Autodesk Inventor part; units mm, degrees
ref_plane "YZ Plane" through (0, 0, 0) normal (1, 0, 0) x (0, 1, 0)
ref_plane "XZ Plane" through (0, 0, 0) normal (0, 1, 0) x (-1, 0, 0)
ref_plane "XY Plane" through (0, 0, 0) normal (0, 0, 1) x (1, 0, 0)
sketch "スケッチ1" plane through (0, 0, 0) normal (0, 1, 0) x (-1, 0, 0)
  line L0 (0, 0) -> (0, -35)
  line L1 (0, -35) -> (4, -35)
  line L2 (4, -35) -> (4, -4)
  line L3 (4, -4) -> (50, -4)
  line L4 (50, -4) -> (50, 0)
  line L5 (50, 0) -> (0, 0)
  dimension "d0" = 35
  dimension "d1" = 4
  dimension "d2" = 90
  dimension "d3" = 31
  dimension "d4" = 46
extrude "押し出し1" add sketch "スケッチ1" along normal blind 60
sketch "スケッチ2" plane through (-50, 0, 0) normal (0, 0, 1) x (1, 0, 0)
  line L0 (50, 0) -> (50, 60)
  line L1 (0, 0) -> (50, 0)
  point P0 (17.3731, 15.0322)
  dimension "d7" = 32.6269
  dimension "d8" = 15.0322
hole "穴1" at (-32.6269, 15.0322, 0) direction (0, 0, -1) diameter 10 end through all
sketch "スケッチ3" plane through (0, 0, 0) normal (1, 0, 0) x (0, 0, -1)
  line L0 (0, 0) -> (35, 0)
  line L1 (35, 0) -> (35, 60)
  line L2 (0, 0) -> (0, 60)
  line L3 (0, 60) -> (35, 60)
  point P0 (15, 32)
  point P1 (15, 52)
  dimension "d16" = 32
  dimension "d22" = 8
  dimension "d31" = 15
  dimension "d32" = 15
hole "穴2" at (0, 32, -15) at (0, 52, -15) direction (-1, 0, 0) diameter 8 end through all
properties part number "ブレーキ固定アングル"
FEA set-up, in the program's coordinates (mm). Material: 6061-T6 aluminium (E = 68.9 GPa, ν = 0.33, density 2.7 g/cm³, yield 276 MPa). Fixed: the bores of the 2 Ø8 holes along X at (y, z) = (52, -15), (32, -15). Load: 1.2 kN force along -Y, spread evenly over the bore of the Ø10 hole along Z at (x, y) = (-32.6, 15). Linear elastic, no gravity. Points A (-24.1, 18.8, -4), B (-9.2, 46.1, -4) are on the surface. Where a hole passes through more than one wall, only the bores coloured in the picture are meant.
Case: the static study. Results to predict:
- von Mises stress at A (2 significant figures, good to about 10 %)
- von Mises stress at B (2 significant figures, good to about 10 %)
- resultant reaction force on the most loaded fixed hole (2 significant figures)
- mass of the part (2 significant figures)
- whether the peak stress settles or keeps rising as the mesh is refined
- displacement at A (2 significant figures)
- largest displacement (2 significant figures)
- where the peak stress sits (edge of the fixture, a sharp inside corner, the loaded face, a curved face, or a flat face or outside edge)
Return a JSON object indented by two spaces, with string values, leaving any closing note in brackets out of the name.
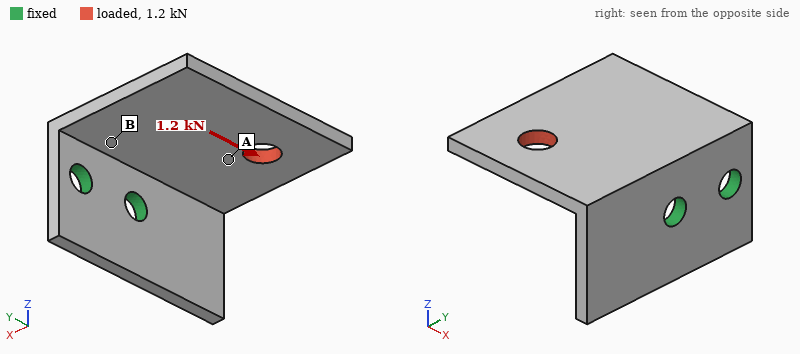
{
  "von Mises stress at A": "27 MPa",
  "von Mises stress at B": "59 MPa",
  "resultant reaction force on the most loaded fixed hole": "1.6 kN",
  "mass of the part": "51 g",
  "whether the peak stress settles or keeps rising as the mesh is refined": "keeps rising",
  "displacement at A": "0.14 mm",
  "largest displacement": "0.31 mm",
  "where the peak stress sits": "edge of the fixture"
}
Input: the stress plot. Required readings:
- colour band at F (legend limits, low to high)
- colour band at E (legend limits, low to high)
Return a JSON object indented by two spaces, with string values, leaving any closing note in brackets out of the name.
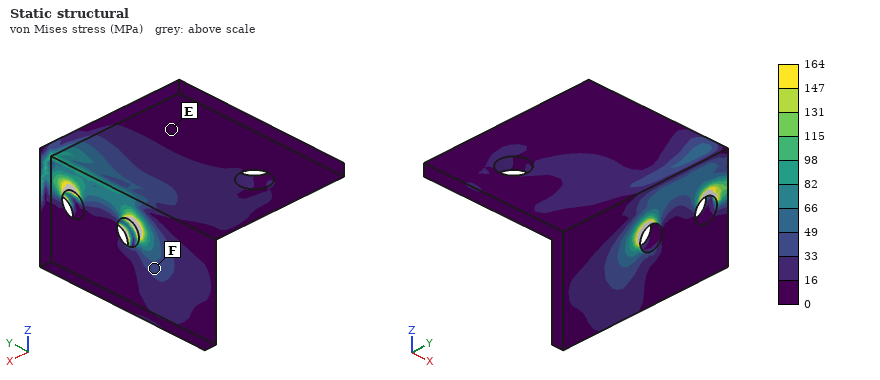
{
  "colour band at F": "33 to 49 MPa",
  "colour band at E": "0 to 16 MPa"
}
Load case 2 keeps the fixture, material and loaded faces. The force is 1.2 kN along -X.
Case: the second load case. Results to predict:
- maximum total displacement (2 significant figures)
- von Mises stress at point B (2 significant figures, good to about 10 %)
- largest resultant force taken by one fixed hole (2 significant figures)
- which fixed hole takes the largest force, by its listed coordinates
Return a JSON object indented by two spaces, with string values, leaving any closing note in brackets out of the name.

{
  "maximum total displacement": "0.39 mm",
  "von Mises stress at point B": "37 MPa",
  "largest resultant force taken by one fixed hole": "1.8 kN",
  "which fixed hole takes the largest force, by its listed coordinates": "(32, -15)"
}
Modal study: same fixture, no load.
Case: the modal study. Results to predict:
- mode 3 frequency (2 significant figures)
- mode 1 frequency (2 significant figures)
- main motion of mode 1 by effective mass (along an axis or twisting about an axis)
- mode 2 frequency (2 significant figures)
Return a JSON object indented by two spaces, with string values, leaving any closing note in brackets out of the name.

{
  "mode 3 frequency": "2900 Hz",
  "mode 1 frequency": "1000 Hz",
  "main motion of mode 1 by effective mass": "along Z",
  "mode 2 frequency": "2300 Hz"
}
